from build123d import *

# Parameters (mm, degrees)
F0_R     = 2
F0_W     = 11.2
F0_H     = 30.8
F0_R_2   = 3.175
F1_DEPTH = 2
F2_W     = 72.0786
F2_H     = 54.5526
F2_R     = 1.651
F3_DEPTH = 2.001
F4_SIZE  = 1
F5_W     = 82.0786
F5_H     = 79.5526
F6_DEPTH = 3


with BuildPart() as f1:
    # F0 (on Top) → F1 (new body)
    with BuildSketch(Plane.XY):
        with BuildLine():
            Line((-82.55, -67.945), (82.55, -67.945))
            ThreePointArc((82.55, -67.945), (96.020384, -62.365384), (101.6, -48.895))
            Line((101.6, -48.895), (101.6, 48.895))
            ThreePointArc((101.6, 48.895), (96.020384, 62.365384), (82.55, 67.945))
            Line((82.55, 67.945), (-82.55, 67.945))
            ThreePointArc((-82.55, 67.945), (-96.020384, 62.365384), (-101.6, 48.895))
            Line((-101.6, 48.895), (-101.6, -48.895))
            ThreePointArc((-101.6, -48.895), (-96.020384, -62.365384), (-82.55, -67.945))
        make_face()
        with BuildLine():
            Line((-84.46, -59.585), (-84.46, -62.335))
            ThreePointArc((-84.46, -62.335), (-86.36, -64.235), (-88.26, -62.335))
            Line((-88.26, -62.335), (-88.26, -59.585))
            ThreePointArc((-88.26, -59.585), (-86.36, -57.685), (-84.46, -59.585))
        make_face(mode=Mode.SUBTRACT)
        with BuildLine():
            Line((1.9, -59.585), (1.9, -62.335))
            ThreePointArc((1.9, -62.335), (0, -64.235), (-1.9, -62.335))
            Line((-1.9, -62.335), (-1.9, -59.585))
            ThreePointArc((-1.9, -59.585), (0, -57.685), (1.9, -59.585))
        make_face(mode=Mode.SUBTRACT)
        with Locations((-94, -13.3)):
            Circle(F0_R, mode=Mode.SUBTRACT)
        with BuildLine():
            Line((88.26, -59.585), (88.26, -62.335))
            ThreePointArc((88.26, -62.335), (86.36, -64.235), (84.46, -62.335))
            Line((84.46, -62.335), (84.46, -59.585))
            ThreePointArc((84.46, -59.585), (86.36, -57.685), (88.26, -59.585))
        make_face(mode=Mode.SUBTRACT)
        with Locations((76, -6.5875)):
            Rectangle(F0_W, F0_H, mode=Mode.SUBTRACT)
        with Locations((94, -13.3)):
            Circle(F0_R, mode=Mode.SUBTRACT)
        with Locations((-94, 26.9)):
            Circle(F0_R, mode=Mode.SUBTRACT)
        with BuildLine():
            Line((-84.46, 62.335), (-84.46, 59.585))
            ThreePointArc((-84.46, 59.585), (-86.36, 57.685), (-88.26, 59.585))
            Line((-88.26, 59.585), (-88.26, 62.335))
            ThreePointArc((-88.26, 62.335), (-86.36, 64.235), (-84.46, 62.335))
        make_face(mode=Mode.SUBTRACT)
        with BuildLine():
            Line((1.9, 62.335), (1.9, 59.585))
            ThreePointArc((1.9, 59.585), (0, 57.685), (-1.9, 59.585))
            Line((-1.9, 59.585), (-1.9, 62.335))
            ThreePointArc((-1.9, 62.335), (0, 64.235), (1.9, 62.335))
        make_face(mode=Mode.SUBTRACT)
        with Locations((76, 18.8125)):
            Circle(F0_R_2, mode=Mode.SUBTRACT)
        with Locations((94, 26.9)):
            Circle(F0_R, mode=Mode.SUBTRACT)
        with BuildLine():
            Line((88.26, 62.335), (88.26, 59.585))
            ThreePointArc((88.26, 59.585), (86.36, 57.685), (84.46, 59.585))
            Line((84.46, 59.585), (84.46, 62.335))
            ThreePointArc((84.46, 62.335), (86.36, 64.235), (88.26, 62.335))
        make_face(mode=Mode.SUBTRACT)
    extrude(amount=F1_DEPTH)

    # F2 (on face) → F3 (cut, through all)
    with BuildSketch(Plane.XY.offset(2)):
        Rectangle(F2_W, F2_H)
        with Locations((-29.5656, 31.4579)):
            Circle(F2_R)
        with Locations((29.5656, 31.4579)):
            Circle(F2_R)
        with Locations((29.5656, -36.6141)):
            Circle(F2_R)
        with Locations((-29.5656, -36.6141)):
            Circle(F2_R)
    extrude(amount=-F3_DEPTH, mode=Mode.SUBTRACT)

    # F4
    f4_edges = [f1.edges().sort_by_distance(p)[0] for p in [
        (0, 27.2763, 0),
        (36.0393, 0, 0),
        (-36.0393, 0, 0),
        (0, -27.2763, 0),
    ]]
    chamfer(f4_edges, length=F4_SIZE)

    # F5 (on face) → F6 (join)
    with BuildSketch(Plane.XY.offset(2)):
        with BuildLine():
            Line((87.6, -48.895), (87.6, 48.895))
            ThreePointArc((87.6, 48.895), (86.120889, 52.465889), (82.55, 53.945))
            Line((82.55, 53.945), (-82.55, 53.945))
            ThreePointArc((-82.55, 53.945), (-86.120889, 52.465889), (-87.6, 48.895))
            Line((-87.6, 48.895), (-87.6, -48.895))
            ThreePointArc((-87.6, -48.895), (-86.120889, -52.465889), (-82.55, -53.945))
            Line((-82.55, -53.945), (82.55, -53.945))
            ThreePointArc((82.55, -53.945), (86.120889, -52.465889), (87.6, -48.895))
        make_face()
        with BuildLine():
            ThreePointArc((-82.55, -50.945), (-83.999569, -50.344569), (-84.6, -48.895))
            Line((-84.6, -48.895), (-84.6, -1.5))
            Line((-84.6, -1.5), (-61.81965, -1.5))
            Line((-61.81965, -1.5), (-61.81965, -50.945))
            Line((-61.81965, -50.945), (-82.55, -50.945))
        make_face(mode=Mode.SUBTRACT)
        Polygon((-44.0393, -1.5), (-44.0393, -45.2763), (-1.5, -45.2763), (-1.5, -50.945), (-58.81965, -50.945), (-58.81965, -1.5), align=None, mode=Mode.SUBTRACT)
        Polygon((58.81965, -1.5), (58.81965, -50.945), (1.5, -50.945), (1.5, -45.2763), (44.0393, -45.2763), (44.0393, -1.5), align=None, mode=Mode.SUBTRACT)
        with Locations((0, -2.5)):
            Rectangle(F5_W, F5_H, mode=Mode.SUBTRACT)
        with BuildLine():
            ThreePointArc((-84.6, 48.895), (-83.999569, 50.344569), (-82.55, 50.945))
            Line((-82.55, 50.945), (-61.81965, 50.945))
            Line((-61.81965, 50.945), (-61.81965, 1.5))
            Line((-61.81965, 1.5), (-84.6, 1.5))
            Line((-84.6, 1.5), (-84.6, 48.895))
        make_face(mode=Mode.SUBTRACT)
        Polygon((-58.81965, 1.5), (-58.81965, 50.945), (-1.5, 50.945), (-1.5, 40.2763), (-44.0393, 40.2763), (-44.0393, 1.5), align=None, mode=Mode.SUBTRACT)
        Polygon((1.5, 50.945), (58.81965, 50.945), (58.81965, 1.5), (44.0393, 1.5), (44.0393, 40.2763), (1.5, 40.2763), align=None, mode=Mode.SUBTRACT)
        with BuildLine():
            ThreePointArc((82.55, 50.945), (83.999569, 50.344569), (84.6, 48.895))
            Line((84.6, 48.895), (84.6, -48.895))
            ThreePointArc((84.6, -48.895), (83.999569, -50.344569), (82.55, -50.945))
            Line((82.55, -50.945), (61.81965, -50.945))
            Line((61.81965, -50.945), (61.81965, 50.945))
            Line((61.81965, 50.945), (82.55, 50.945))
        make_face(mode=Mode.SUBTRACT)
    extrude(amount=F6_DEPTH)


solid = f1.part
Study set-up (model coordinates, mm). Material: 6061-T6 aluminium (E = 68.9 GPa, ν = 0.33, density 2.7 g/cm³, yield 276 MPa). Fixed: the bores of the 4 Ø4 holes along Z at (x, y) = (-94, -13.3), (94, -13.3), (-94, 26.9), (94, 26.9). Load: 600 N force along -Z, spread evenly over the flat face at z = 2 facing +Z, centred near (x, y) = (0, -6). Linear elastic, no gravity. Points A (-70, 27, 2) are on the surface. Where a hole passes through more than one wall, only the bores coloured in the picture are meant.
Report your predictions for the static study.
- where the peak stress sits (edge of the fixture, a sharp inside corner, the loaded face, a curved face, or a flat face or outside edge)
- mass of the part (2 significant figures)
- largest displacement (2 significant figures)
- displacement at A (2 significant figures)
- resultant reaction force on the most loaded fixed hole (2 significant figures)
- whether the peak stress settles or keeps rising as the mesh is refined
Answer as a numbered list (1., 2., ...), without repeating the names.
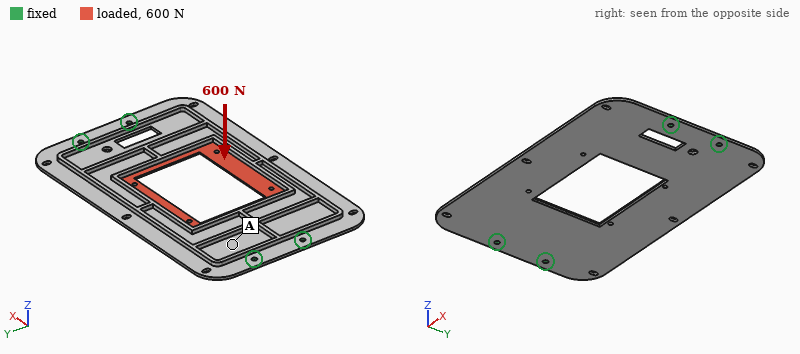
1. edge of the fixture
2. 150 g
3. 2.6 mm
4. 0.46 mm
5. 550 N
6. keeps rising
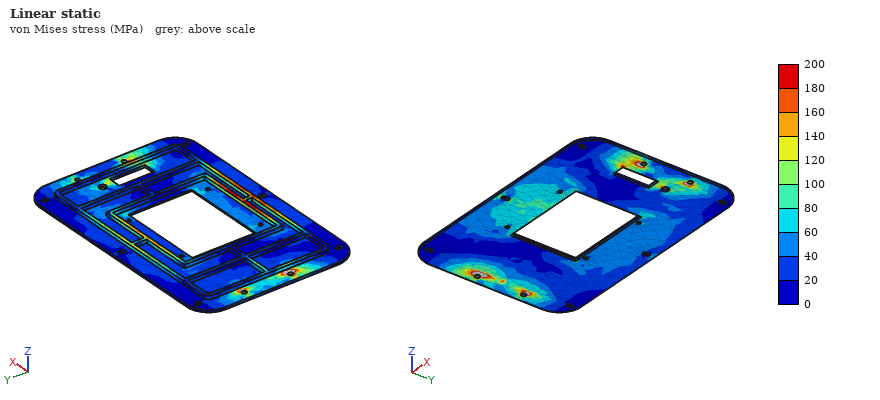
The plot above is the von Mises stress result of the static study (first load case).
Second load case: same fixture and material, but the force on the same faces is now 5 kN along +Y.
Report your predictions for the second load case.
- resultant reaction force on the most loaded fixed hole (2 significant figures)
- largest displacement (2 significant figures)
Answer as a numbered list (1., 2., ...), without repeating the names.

1. 1.5 kN
2. 0.58 mm
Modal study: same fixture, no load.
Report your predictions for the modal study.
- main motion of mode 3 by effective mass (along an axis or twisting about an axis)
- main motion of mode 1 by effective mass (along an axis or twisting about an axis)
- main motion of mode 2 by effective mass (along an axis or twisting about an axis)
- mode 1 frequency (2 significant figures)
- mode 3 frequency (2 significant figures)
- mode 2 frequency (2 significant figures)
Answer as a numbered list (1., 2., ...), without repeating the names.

1. twisting about Y
2. along Z
3. along Z
4. 320 Hz
5. 720 Hz
6. 380 Hz
